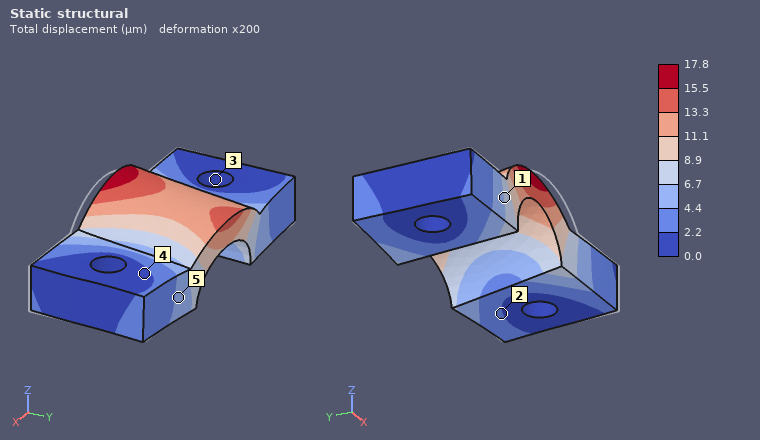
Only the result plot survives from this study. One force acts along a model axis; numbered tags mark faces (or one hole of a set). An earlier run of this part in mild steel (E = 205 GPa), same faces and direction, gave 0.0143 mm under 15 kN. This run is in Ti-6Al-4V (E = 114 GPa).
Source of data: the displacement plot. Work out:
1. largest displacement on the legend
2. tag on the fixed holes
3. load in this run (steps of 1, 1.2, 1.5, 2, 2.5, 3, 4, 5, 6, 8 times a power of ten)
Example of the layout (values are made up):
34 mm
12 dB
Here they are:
17.8 µm
3
10 kN
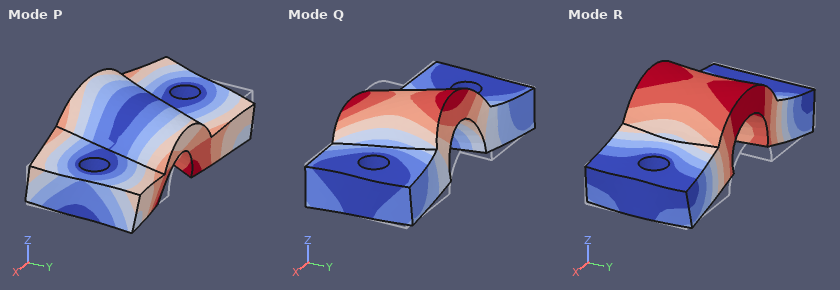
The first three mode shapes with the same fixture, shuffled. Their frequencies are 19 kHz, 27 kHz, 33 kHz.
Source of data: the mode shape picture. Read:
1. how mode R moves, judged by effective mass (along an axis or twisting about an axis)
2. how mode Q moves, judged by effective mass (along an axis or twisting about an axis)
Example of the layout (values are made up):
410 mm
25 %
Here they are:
along Z
along Y
